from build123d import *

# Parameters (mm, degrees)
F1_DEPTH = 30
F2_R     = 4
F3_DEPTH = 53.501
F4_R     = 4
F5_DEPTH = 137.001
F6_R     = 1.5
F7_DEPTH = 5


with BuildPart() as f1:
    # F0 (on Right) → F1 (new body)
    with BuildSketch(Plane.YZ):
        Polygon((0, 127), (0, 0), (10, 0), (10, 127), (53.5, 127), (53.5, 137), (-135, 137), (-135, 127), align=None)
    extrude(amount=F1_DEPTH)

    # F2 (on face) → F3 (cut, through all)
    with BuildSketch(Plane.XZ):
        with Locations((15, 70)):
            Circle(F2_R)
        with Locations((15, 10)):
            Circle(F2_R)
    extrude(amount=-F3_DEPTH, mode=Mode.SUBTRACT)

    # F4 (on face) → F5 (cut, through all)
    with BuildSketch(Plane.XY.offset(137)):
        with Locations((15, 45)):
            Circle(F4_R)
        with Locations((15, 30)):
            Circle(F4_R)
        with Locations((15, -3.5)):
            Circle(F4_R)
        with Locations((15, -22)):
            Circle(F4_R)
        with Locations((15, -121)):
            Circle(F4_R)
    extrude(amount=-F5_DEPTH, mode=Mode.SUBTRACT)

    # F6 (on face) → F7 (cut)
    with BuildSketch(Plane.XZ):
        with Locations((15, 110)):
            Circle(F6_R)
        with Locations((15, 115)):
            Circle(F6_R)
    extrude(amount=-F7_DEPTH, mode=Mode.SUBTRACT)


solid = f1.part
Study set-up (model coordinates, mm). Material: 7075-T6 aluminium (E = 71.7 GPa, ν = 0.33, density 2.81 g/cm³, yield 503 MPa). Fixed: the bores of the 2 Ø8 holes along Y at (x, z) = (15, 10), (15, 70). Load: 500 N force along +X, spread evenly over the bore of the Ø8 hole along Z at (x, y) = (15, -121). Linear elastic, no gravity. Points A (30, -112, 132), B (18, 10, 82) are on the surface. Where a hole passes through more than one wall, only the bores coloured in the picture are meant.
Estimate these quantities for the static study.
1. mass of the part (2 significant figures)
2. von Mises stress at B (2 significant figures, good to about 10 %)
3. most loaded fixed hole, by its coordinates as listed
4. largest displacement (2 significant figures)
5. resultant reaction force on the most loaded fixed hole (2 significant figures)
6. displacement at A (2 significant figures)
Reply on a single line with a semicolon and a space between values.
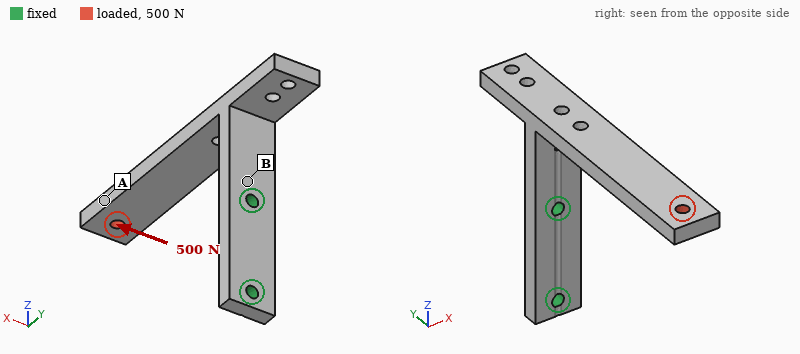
260 g; 110 MPa; (15, 70); 2.6 mm; 810 N; 2.1 mm
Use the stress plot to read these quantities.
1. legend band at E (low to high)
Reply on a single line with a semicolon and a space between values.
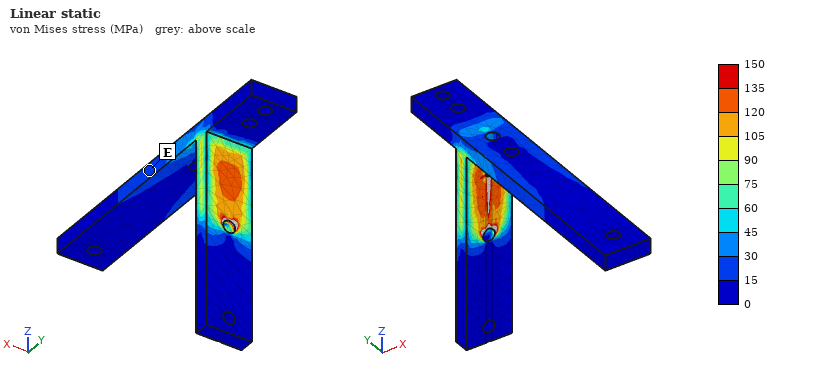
15 to 30 MPa
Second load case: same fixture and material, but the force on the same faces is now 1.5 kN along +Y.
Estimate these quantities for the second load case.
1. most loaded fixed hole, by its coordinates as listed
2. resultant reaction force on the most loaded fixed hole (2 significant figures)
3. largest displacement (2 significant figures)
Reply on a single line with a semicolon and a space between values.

(15, 70); 1.7 kN; 2.3 mm
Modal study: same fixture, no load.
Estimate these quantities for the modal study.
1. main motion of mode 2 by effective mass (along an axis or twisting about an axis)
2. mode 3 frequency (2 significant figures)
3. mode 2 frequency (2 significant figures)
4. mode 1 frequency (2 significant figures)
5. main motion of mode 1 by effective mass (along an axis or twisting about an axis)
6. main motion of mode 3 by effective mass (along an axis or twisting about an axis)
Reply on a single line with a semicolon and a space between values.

along X; 820 Hz; 340 Hz; 240 Hz; along Z; along Y
